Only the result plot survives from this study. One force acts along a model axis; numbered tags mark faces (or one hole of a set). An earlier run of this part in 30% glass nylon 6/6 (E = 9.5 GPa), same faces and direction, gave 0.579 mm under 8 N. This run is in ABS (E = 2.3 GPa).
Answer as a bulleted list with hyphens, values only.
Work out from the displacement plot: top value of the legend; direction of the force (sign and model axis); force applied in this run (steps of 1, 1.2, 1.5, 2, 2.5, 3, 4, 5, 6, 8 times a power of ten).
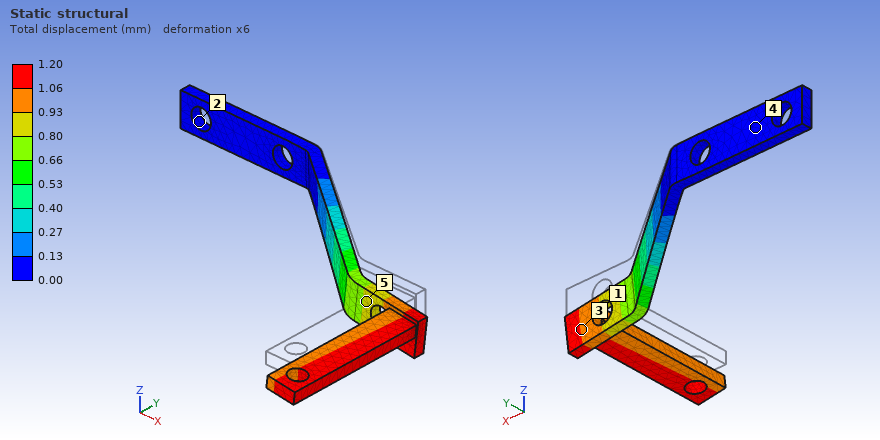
- 1.20 mm
- -Z
- 4 N
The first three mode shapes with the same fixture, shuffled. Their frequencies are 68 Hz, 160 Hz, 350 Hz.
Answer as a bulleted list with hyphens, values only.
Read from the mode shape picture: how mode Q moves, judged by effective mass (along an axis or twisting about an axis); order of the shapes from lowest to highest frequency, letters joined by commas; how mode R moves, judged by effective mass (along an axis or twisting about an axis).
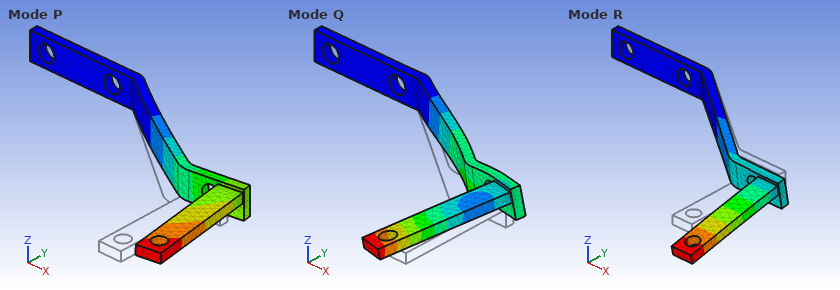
- along Y
- P, R, Q
- along Z
